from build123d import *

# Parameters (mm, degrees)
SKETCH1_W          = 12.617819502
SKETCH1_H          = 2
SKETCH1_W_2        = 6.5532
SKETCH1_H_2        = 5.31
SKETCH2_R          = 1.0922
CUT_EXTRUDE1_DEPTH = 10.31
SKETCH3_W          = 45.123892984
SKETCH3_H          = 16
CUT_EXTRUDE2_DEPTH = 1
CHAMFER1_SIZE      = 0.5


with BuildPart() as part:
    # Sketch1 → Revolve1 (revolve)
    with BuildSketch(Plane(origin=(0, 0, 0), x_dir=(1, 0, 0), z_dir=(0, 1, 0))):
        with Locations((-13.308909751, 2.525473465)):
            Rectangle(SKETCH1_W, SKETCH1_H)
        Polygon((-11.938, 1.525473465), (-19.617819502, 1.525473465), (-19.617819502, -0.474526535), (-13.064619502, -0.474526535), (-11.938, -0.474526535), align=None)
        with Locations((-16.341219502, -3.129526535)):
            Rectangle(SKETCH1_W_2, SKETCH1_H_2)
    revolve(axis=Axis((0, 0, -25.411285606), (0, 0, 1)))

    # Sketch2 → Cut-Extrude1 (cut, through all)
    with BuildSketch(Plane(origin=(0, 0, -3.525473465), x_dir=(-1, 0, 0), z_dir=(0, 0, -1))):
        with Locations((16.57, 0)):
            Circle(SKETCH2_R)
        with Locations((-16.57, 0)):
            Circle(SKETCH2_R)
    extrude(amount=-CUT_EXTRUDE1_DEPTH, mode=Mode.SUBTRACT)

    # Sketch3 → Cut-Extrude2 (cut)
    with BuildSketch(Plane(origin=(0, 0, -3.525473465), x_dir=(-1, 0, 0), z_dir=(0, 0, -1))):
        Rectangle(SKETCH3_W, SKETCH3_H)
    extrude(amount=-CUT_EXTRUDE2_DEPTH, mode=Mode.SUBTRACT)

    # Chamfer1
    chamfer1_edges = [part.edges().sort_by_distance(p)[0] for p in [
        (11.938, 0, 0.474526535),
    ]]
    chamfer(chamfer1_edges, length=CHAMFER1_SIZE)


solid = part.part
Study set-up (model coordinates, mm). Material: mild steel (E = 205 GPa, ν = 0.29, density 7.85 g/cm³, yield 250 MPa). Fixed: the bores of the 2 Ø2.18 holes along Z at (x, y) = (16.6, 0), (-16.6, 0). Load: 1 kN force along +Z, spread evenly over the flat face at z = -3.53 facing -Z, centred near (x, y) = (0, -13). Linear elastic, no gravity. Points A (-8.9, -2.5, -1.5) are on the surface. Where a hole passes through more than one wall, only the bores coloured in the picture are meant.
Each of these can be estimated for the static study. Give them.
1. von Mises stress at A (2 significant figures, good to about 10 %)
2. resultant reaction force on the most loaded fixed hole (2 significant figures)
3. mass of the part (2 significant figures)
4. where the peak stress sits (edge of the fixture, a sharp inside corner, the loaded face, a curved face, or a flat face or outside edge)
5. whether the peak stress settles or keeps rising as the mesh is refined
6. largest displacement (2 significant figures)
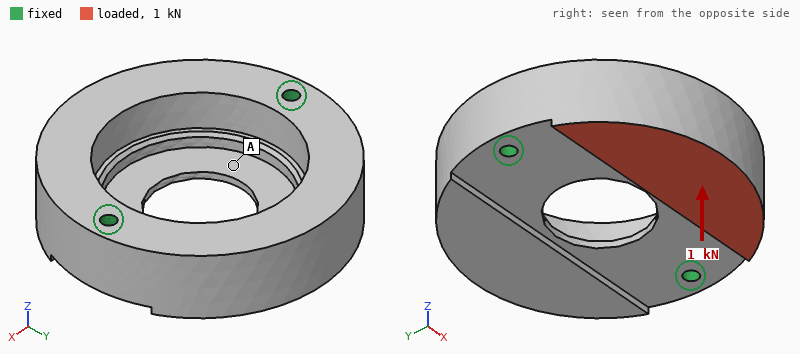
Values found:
12 MPa
530 N
52 g
edge of the fixture
keeps rising
14 µm
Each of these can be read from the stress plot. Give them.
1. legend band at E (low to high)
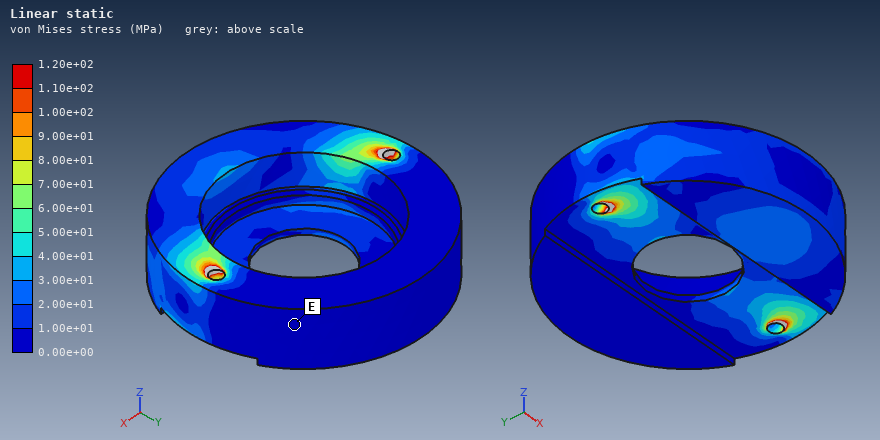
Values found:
0.00e+00 to 1.00e+01 MPa
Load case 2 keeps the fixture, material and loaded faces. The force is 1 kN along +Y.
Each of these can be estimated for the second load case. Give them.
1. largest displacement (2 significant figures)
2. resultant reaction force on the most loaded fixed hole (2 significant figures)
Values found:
7.2 µm
530 N
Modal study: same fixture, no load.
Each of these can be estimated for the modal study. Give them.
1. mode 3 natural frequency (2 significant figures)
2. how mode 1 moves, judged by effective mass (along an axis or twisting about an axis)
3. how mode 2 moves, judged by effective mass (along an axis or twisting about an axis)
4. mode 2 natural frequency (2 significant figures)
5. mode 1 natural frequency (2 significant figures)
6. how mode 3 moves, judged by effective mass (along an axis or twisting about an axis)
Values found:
20 kHz
twisting about X
along Z
12 kHz
11 kHz
twisting about Z
